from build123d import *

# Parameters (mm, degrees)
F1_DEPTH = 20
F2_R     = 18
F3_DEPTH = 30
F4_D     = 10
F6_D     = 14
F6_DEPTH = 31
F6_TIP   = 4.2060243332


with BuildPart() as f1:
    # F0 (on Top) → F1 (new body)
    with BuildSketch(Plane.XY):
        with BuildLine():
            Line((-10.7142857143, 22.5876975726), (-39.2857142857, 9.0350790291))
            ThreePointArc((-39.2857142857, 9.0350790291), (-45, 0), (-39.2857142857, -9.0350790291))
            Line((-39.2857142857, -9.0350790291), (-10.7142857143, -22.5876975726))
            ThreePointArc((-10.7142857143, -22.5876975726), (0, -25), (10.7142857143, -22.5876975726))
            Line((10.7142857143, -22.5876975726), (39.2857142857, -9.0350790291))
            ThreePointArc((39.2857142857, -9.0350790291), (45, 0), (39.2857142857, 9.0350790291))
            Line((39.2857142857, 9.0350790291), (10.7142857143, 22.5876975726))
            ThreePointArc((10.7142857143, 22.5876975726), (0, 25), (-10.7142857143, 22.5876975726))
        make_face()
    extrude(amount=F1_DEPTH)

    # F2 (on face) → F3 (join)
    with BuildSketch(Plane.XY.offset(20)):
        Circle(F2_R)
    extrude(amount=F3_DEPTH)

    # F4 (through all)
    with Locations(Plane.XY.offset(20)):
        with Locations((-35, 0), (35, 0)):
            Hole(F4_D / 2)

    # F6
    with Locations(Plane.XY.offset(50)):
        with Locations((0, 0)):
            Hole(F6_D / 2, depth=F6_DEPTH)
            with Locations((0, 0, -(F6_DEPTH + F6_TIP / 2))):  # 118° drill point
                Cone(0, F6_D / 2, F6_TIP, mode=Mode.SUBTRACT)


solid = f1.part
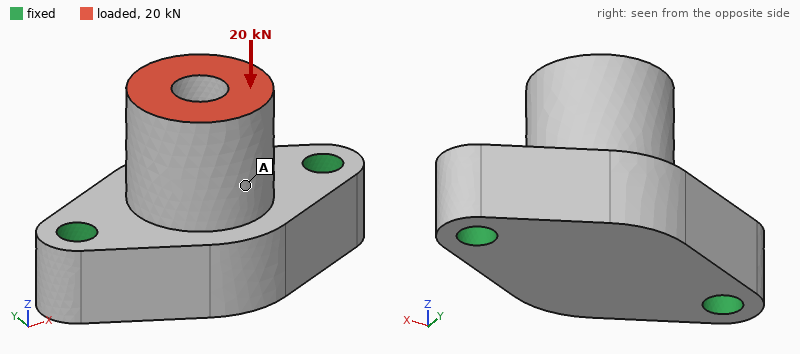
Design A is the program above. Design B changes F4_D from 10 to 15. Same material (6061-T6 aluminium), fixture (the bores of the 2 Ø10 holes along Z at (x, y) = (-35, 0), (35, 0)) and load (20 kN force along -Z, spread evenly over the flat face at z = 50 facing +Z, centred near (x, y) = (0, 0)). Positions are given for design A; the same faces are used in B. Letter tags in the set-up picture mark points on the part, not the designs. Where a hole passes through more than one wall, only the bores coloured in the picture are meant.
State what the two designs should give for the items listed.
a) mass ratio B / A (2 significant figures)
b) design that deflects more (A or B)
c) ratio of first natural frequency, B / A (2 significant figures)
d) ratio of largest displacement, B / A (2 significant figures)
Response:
0.95
A
1.1
0.83
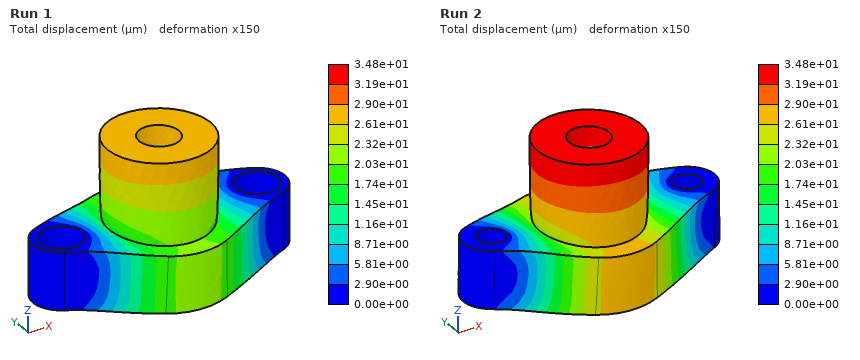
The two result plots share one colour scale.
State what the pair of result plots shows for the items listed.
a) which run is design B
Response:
Run 1
